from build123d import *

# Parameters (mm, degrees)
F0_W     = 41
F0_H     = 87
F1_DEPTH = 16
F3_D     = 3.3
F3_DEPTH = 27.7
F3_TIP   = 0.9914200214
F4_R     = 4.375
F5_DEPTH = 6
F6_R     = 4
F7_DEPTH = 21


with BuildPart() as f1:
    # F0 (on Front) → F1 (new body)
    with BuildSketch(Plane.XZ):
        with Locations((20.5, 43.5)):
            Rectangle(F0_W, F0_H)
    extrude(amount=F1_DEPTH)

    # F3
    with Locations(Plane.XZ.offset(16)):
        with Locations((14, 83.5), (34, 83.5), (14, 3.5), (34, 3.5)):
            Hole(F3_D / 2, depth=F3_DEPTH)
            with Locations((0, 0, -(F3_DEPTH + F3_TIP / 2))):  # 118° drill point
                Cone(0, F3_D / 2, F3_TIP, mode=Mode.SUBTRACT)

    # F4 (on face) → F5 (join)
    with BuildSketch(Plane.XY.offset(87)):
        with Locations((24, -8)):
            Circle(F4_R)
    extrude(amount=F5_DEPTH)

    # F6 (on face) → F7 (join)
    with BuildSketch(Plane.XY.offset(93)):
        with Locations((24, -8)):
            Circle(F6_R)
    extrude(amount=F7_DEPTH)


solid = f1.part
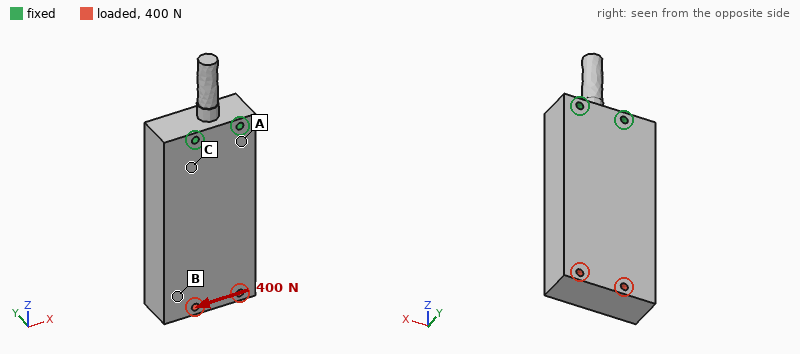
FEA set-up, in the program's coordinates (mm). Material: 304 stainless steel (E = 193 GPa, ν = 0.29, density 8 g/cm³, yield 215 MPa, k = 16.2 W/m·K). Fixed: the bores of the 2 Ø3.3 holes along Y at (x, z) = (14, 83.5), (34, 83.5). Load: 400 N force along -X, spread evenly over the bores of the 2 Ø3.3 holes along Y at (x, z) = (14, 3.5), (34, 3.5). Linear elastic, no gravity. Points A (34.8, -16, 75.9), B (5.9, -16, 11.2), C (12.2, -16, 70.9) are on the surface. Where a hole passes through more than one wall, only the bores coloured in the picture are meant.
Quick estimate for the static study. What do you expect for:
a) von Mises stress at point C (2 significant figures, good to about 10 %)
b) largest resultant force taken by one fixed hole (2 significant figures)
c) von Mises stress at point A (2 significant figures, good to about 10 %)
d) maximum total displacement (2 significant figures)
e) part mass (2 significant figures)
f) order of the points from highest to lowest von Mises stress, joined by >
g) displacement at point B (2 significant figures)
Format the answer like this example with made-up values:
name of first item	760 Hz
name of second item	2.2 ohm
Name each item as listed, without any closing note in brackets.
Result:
von Mises stress at point C	4.7 MPa
largest resultant force taken by one fixed hole	1.5 kN
von Mises stress at point A	7.0 MPa
maximum total displacement	7.7 µm
part mass	460 g
order of the points from highest to lowest von Mises stress, joined by >	A > C > B
displacement at point B	6.4 µm
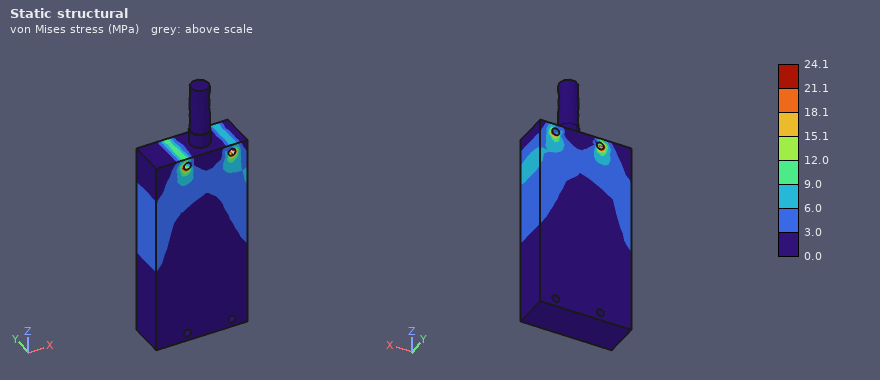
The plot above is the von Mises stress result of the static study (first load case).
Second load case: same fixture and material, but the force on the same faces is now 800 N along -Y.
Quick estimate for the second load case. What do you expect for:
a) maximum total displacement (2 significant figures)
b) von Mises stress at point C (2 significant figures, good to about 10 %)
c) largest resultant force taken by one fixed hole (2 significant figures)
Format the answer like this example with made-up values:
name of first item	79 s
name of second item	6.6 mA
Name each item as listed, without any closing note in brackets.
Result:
maximum total displacement	67 µm
von Mises stress at point C	31 MPa
largest resultant force taken by one fixed hole	410 N
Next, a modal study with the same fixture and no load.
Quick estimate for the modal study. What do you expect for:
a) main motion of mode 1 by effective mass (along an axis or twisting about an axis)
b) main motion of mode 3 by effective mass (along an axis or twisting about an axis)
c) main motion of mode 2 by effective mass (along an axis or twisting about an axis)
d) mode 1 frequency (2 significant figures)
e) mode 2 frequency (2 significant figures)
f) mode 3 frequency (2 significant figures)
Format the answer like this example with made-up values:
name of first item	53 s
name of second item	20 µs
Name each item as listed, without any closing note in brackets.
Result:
main motion of mode 1 by effective mass	along Y
main motion of mode 3 by effective mass	twisting about Z
main motion of mode 2 by effective mass	along X
mode 1 frequency	1600 Hz
mode 2 frequency	3100 Hz
mode 3 frequency	6000 Hz
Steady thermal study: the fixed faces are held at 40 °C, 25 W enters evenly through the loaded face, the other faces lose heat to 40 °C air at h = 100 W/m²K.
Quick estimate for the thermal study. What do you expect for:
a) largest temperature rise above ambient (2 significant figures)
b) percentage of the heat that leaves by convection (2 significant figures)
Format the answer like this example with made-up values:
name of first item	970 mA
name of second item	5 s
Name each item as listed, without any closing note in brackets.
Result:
largest temperature rise above ambient	71 K
percentage of the heat that leaves by convection	90 %
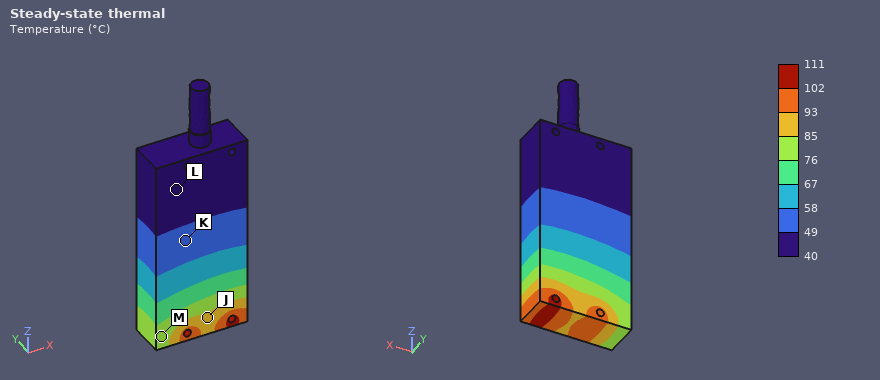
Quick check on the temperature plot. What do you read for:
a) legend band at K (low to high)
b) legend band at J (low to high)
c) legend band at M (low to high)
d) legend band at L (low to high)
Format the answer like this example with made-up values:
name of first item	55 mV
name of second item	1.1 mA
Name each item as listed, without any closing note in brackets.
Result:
legend band at K	49 to 58 °C
legend band at J	85 to 93 °C
legend band at M	76 to 85 °C
legend band at L	40 to 49 °C
